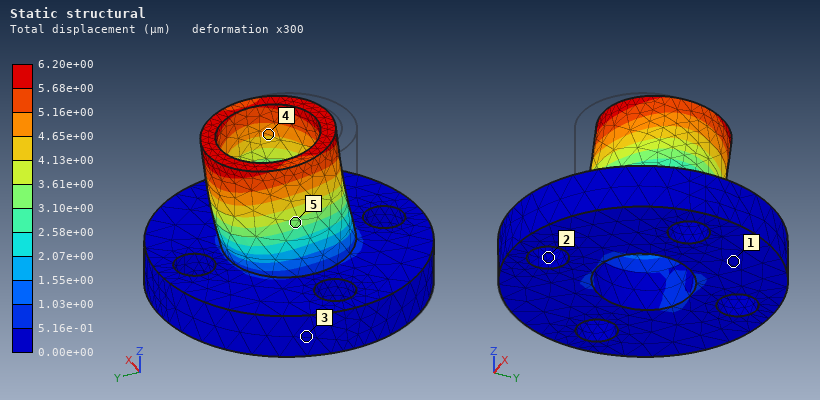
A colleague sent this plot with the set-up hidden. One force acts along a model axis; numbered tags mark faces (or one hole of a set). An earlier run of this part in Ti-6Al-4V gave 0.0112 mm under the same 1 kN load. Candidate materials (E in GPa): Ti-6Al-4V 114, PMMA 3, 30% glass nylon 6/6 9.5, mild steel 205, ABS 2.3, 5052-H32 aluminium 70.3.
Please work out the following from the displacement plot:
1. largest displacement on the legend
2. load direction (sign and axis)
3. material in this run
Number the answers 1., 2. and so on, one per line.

1. 6.20e+00 µm
2. +Y
3. mild steel
